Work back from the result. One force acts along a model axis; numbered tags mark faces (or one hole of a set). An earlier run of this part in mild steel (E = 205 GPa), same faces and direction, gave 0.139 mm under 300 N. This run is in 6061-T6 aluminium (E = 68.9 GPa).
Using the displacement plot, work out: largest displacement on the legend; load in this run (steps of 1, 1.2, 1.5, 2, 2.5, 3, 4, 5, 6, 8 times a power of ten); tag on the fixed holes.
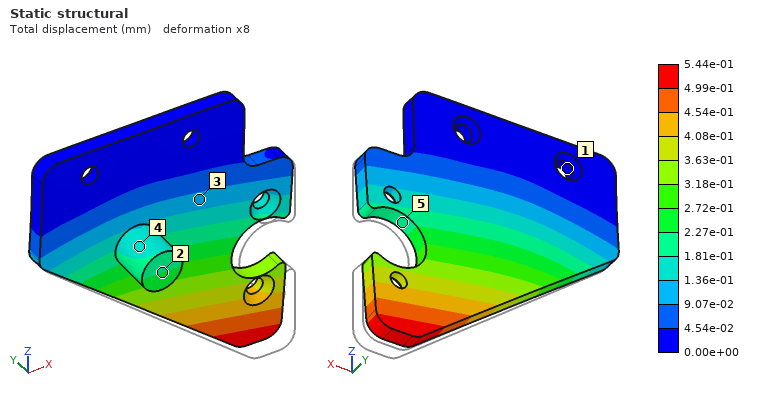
5.44e-01 mm
400 N
1
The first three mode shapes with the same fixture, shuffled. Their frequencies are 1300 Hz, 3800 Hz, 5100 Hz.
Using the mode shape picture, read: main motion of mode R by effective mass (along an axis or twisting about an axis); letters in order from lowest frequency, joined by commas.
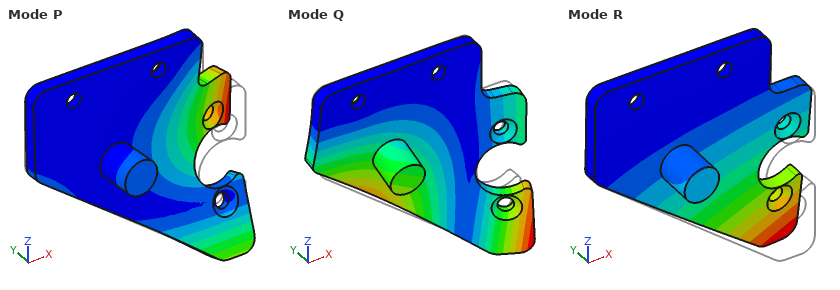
along Y
R, Q, P
